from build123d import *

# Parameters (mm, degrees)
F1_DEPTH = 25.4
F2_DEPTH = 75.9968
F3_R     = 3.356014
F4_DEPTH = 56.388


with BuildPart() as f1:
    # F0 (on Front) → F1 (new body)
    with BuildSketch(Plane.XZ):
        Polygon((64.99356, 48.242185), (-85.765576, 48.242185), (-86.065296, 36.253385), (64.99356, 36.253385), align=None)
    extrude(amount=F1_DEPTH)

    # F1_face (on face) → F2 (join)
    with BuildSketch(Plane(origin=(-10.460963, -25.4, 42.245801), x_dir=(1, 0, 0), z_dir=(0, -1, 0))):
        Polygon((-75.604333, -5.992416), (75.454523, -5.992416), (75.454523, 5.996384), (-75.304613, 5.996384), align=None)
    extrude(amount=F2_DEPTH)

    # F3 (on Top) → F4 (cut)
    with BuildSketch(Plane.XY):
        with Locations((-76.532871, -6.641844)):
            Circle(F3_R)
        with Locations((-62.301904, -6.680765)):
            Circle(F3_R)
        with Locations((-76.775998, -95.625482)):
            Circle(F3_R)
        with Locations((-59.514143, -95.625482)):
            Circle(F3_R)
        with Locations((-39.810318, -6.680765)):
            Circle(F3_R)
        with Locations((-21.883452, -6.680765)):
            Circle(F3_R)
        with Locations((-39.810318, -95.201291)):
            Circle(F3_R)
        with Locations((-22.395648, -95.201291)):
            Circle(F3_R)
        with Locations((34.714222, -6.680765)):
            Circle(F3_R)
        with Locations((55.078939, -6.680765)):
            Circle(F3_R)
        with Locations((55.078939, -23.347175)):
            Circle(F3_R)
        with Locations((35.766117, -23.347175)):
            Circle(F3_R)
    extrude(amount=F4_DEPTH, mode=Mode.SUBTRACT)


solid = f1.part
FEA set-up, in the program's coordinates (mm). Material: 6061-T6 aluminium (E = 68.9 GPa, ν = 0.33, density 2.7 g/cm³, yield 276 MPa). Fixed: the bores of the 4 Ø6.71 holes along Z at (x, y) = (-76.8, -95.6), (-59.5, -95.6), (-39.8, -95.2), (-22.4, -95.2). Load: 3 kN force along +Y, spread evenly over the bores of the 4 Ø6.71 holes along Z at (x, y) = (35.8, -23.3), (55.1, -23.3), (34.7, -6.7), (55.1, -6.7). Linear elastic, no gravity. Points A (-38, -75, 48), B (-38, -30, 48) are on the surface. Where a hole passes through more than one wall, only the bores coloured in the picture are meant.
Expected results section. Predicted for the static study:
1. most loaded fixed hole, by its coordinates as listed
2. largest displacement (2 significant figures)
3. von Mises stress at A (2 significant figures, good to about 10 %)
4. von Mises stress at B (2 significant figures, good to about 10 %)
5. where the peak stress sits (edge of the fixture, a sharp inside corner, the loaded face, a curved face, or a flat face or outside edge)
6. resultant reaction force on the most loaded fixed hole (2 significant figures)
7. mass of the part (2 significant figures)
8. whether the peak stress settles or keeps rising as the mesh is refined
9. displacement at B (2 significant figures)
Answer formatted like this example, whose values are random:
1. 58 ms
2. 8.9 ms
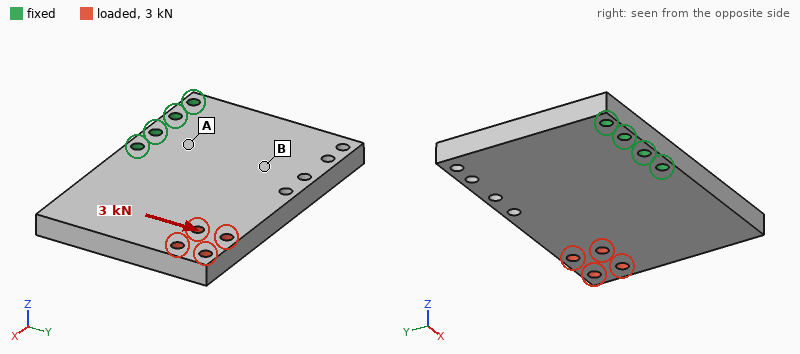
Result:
1. (-22.4, -95.2)
2. 68 µm
3. 10 MPa
4. 5.5 MPa
5. edge of the fixture
6. 6.1 kN
7. 480 g
8. keeps rising
9. 23 µm
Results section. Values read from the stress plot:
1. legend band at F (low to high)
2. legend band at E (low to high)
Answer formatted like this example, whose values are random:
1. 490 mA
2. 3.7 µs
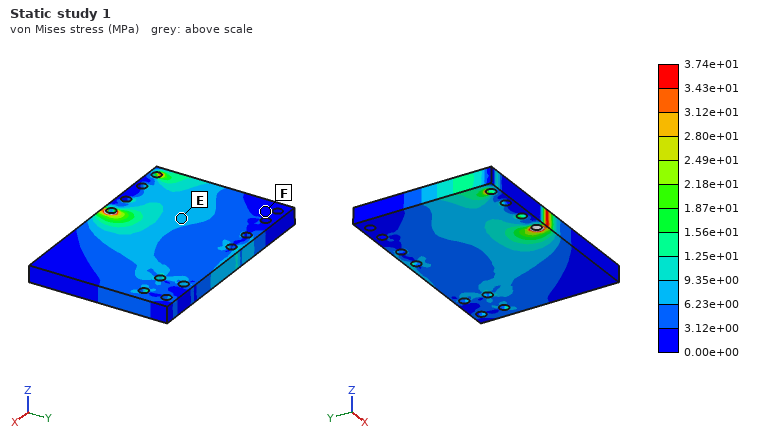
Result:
1. 0.00e+00 to 3.12e+00 MPa
2. 6.23e+00 to 9.35e+00 MPa
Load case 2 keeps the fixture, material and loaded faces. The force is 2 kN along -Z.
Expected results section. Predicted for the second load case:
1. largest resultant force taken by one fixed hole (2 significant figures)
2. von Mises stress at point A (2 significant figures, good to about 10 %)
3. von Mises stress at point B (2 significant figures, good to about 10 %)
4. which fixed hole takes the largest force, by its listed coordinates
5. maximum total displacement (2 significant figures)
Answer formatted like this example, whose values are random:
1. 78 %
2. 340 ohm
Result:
1. 3.4 kN
2. 71 MPa
3. 43 MPa
4. (-22.4, -95.2)
5. 1.4 mm
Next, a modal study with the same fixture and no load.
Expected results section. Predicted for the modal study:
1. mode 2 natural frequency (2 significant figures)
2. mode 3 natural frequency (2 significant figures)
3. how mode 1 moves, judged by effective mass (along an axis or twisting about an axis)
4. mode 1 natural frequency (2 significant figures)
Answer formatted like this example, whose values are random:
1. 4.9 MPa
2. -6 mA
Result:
1. 1200 Hz
2. 2400 Hz
3. along Z
4. 700 Hz
